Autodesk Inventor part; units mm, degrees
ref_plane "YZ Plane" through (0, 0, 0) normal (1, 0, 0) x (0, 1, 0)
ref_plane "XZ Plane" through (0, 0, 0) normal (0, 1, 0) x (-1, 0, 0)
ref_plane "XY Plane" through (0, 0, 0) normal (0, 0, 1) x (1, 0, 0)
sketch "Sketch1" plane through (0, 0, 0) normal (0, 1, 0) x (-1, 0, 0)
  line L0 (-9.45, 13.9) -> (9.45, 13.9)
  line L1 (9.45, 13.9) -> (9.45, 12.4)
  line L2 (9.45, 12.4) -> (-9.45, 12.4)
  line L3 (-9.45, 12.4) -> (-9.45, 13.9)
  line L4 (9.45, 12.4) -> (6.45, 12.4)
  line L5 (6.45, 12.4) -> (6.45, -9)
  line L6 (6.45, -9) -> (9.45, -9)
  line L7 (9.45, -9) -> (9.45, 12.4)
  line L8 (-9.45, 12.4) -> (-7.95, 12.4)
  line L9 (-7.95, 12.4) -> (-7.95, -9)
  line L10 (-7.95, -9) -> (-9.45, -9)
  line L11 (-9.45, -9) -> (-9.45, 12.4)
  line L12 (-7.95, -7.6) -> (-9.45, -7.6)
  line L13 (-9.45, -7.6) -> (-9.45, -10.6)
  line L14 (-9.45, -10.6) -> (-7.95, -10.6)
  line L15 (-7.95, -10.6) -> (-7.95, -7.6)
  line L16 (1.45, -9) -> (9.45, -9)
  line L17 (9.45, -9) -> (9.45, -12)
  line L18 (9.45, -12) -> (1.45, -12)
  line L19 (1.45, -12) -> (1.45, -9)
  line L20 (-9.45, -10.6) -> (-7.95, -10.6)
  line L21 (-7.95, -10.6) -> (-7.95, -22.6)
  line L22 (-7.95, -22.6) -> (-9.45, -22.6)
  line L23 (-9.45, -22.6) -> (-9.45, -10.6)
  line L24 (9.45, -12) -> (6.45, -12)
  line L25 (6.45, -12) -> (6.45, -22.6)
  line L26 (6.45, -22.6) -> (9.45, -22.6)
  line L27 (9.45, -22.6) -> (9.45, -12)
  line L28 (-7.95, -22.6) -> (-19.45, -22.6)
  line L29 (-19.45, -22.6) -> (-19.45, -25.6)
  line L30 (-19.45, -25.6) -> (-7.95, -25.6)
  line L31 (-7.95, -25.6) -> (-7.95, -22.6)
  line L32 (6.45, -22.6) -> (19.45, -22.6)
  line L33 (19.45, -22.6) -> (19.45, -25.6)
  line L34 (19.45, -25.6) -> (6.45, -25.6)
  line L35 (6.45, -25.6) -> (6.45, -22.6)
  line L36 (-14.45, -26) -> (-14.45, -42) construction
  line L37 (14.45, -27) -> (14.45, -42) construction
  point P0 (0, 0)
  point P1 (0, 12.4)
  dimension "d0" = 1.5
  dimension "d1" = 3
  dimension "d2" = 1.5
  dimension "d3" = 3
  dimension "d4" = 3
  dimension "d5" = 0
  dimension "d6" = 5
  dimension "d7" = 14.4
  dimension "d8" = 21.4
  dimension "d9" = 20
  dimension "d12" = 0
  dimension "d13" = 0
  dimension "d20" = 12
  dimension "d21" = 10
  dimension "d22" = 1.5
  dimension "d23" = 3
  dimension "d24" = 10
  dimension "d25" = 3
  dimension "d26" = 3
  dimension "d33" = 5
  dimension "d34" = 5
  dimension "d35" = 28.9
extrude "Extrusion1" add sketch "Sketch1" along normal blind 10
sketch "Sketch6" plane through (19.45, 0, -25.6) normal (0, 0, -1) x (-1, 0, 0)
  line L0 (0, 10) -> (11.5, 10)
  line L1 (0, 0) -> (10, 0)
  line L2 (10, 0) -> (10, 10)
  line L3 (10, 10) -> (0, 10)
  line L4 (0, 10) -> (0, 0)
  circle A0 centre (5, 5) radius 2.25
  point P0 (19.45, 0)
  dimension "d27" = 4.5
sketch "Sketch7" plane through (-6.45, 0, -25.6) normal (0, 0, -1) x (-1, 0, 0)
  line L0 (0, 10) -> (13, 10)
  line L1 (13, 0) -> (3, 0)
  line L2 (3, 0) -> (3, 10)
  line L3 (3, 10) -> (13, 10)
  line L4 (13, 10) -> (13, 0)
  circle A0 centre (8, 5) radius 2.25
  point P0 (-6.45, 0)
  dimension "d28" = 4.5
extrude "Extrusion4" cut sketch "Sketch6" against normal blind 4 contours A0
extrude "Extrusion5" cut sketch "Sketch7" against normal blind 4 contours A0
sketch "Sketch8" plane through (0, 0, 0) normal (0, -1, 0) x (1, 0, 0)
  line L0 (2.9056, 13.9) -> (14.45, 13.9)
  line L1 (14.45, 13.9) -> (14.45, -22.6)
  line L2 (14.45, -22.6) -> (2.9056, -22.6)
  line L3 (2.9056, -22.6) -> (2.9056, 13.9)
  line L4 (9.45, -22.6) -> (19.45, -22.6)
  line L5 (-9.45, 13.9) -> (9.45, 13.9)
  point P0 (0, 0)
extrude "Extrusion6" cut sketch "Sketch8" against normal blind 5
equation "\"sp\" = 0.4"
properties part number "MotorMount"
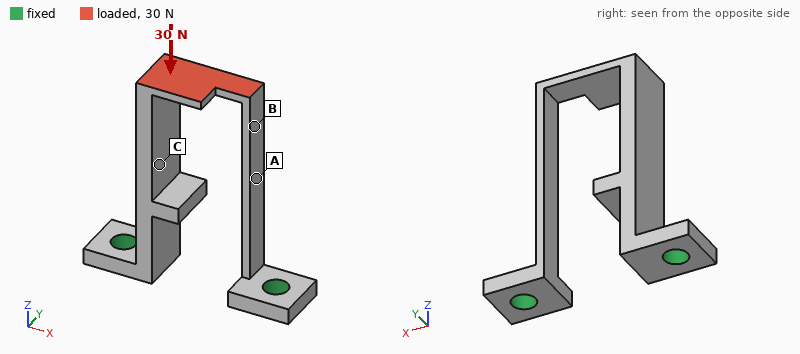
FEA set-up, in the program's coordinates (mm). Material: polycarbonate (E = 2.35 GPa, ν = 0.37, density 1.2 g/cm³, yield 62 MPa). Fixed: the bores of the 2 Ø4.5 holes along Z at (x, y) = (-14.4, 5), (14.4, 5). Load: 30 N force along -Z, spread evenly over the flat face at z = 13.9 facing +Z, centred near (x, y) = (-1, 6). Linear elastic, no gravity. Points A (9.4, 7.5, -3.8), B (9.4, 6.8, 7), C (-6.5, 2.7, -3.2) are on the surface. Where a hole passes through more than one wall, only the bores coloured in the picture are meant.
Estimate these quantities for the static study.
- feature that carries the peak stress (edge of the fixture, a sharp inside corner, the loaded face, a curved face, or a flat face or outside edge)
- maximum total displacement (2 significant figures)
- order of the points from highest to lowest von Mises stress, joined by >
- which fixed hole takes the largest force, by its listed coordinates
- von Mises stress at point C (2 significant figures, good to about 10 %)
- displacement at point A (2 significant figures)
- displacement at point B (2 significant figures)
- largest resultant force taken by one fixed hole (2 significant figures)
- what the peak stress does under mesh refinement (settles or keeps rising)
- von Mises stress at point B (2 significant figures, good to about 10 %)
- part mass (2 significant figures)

a sharp inside corner
0.54 mm
B > C > A
(-14.4, 5)
2.4 MPa
0.36 mm
0.51 mm
19 N
keeps rising
4.7 MPa
2.8 g
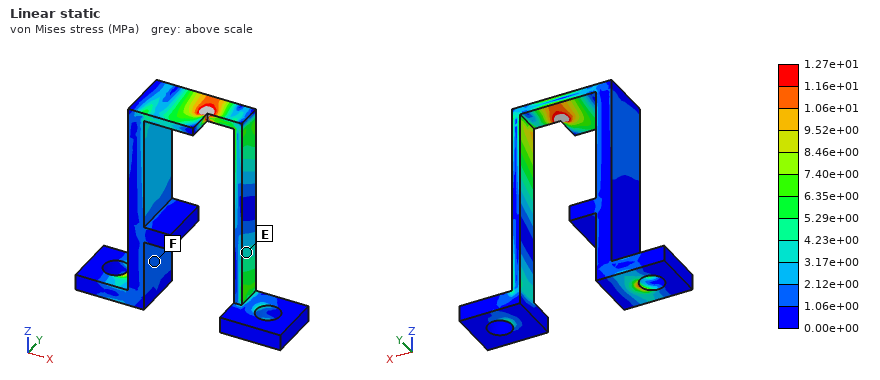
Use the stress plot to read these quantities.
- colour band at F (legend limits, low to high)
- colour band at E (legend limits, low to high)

1.06e+00 to 2.12e+00 MPa
3.17e+00 to 4.23e+00 MPa
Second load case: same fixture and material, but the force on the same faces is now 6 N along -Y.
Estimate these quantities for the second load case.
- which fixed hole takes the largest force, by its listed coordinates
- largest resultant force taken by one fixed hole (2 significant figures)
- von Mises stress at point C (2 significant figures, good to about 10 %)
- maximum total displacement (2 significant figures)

(-14.4, 5)
4.9 N
1.9 MPa
0.63 mm
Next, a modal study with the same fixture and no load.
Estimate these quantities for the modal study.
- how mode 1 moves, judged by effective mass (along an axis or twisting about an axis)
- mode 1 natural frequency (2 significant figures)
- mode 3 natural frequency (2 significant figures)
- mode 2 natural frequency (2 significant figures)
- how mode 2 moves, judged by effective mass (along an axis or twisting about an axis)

along X
410 Hz
1300 Hz
630 Hz
along Y
